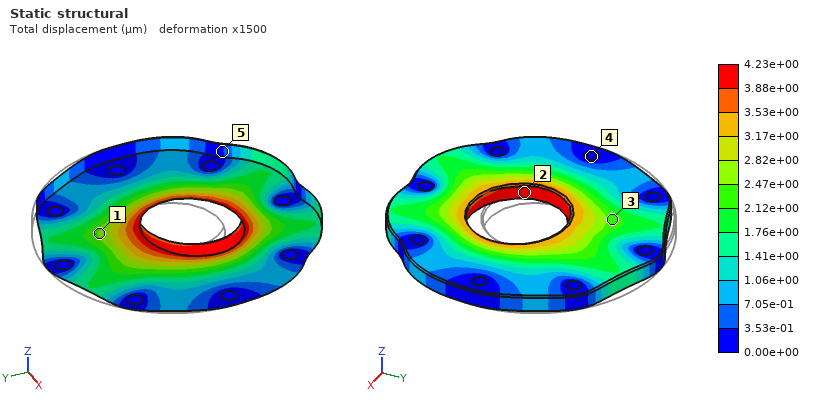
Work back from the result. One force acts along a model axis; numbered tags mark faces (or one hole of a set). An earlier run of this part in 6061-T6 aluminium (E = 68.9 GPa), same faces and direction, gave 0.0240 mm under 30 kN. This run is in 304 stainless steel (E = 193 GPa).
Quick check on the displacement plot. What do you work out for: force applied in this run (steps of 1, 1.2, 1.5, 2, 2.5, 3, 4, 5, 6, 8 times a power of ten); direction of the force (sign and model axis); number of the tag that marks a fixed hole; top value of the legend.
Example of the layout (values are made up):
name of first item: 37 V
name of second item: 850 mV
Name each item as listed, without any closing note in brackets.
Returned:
force applied in this run: 15 kN
direction of the force: -Y
number of the tag that marks a fixed hole: 4
top value of the legend: 4.23e+00 µm
